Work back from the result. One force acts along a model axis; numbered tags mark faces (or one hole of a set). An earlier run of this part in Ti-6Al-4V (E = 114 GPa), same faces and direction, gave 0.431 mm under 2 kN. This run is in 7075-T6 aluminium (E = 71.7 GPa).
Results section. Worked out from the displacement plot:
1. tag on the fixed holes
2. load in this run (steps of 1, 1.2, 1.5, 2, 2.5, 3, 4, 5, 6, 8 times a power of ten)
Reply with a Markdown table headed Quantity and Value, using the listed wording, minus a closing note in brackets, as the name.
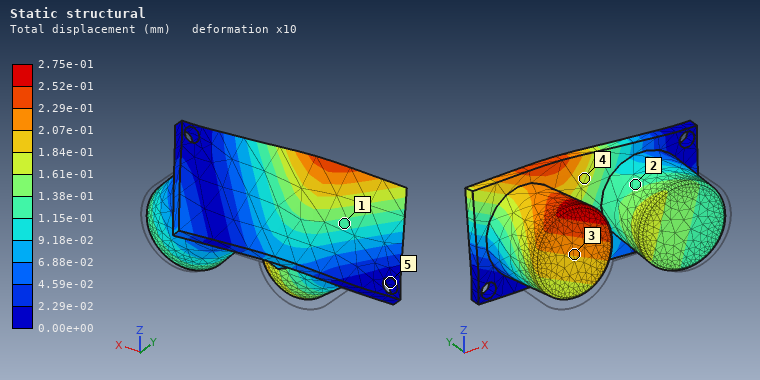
| Quantity | Value |
|---|---|
| tag on the fixed holes | 5 |
| load in this run | 800 N |
